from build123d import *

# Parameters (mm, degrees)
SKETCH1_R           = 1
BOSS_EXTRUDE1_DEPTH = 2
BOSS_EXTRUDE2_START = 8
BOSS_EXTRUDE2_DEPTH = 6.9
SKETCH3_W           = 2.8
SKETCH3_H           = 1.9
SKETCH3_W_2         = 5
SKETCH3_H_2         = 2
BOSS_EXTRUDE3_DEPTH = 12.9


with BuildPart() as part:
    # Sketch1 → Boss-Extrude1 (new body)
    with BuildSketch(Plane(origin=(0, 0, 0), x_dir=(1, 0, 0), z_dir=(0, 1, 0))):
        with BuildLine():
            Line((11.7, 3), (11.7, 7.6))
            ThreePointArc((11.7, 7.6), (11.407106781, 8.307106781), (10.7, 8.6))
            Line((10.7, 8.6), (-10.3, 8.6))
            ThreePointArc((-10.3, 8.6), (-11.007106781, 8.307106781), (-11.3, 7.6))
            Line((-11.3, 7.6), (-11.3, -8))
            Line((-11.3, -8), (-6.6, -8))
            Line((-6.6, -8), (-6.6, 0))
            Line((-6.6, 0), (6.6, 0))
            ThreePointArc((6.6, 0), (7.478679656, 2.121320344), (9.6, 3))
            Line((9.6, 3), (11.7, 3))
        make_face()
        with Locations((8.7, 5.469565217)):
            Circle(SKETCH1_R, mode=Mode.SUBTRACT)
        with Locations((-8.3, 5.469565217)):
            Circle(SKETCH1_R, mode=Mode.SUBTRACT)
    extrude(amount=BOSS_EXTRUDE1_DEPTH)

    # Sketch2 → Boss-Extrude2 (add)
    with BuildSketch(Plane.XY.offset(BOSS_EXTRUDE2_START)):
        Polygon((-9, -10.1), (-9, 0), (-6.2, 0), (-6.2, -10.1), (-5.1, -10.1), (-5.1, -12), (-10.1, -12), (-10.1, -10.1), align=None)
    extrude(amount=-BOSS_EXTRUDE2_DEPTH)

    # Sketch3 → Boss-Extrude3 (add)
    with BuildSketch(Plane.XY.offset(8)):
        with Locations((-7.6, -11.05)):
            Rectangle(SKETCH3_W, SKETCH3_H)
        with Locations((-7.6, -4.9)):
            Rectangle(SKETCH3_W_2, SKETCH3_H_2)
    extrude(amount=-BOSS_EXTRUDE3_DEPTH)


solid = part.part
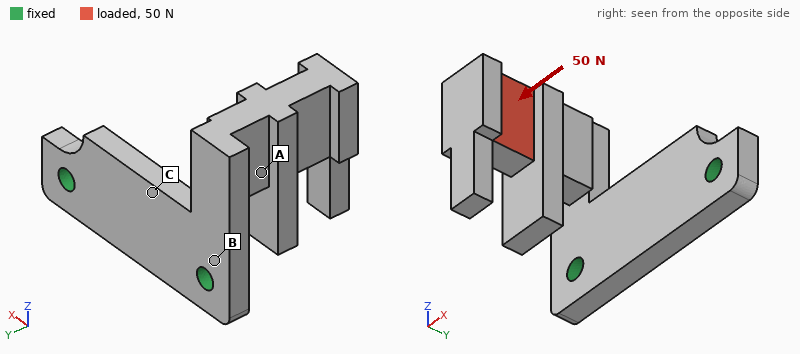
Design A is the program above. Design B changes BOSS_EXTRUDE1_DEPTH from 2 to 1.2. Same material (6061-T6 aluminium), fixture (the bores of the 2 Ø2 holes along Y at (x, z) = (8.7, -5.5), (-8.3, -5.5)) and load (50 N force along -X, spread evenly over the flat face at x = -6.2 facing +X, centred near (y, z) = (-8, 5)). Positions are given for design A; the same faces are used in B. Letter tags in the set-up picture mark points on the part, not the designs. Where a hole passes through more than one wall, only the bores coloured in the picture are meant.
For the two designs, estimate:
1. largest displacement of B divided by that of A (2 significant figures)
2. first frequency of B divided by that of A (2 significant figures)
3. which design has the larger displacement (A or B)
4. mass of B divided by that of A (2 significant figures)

2.8
0.52
B
0.79
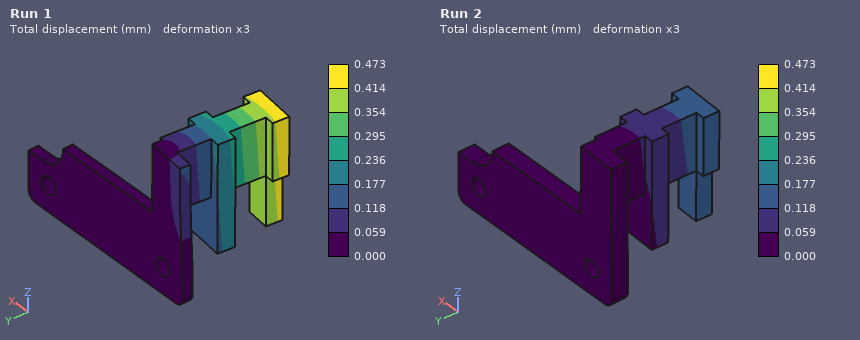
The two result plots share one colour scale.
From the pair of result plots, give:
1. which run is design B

Run 1
